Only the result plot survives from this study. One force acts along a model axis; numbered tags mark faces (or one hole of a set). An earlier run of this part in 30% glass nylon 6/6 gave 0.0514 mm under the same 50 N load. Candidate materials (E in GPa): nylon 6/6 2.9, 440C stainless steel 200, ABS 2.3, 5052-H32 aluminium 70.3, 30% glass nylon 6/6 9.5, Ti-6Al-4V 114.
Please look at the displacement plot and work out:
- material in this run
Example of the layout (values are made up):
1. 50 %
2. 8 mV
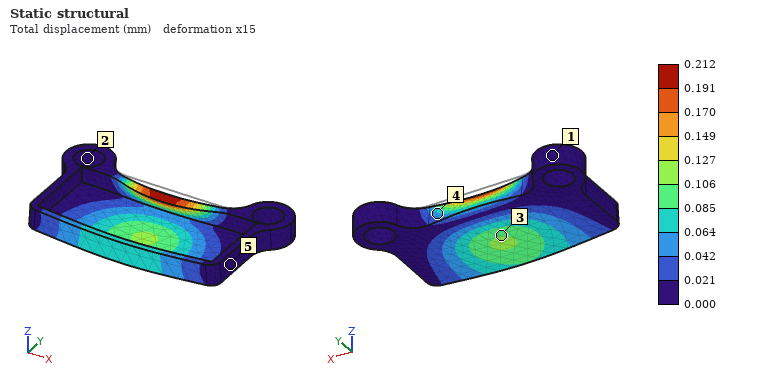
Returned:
1. ABS
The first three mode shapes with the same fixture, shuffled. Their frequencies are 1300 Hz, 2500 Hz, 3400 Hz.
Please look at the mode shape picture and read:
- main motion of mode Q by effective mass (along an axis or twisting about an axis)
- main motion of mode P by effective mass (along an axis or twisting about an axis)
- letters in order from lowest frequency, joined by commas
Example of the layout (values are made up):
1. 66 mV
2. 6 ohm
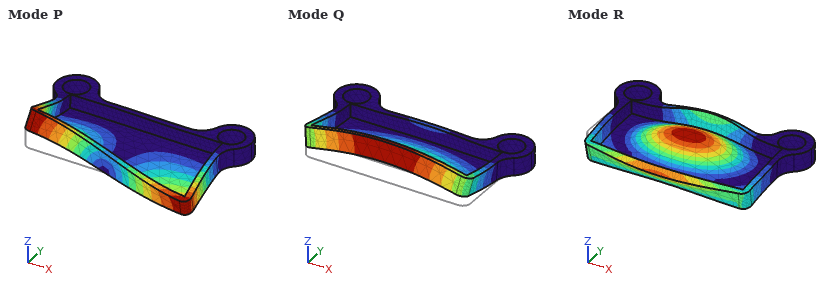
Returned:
1. along Z
2. twisting about Y
3. Q, P, R
